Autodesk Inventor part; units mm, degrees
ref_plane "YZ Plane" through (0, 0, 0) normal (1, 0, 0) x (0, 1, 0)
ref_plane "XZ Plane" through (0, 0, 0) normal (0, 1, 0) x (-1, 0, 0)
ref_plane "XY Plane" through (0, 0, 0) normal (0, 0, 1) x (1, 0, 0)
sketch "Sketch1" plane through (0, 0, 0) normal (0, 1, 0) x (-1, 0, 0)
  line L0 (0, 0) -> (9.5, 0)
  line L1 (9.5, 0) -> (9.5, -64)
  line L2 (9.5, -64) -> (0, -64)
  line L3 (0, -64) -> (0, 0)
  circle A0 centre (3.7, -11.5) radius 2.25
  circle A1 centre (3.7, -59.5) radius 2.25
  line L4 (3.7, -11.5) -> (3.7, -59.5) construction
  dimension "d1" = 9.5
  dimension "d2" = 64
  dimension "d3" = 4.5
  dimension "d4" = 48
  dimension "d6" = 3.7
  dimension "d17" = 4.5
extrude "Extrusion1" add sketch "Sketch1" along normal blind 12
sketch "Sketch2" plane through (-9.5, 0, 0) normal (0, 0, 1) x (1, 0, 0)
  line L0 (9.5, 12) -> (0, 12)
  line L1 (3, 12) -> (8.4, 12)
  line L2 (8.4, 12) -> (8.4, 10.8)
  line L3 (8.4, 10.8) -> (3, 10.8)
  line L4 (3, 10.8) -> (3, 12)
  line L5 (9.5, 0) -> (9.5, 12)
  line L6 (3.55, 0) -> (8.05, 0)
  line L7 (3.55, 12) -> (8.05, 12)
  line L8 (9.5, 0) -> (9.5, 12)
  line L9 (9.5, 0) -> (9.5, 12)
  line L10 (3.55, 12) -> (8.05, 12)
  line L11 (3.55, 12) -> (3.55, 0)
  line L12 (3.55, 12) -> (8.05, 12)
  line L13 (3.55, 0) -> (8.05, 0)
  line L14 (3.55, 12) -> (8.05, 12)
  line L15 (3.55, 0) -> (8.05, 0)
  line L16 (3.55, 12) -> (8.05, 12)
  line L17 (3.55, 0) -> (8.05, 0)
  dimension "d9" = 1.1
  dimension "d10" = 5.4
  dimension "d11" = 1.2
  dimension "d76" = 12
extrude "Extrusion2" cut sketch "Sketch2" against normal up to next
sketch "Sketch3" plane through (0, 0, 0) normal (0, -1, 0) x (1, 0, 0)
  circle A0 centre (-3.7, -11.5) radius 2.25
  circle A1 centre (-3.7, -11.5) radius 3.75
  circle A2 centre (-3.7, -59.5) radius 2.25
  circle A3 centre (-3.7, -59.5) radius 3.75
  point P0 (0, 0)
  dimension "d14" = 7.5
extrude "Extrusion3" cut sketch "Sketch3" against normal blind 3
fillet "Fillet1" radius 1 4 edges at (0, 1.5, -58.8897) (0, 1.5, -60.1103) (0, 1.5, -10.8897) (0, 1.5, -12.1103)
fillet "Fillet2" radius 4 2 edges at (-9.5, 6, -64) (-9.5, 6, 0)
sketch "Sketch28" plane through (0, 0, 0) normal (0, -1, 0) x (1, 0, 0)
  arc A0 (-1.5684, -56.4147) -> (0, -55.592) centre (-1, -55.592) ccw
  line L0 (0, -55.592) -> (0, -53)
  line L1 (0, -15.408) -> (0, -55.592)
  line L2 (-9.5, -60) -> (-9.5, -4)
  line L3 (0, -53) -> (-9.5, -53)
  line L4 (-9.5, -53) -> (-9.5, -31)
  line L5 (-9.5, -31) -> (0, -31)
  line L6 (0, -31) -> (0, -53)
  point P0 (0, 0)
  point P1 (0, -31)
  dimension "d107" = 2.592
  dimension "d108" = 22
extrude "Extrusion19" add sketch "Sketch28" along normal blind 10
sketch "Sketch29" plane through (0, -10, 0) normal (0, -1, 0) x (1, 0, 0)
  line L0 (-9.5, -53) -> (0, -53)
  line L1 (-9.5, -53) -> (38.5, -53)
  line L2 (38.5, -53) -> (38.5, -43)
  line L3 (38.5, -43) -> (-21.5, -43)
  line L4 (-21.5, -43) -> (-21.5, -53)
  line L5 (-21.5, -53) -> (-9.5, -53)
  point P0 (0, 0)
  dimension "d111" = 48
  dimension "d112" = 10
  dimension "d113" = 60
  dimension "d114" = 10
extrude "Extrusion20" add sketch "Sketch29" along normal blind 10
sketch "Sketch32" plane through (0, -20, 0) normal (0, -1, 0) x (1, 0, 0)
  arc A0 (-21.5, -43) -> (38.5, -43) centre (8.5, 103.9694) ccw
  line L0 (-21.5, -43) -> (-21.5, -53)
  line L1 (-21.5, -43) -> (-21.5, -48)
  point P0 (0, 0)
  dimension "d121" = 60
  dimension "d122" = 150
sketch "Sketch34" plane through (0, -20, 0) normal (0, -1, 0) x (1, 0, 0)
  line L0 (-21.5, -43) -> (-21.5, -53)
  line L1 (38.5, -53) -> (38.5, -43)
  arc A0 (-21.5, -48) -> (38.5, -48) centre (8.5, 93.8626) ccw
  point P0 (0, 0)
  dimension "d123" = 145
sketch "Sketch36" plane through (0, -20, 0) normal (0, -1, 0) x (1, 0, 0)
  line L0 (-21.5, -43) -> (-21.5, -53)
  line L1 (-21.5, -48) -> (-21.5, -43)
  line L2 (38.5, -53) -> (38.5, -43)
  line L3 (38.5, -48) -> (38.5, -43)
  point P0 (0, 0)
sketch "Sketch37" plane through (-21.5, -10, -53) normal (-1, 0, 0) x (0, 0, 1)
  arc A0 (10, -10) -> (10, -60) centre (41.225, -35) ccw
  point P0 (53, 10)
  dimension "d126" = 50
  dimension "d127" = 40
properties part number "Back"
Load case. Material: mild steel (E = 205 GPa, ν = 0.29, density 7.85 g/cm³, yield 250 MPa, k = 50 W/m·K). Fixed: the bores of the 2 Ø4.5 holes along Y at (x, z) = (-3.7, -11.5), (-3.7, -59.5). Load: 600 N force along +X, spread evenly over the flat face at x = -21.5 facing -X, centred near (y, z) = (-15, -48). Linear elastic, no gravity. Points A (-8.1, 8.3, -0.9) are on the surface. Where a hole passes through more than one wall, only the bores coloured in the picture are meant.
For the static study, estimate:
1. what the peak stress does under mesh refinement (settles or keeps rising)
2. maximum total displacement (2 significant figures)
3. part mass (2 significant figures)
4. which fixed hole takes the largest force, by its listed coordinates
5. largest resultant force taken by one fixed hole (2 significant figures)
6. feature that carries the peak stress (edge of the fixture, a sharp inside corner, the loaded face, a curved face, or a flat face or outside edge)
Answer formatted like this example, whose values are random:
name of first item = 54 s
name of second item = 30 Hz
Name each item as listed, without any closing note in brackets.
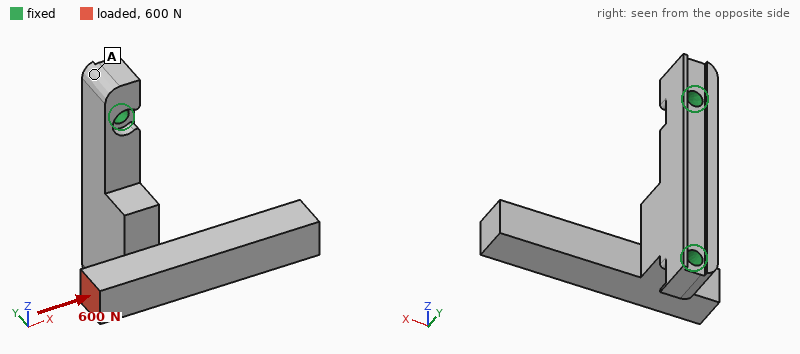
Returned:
what the peak stress does under mesh refinement = keeps rising
maximum total displacement = 63 µm
part mass = 110 g
which fixed hole takes the largest force, by its listed coordinates = (-3.7, -59.5)
largest resultant force taken by one fixed hole = 500 N
feature that carries the peak stress = edge of the fixture
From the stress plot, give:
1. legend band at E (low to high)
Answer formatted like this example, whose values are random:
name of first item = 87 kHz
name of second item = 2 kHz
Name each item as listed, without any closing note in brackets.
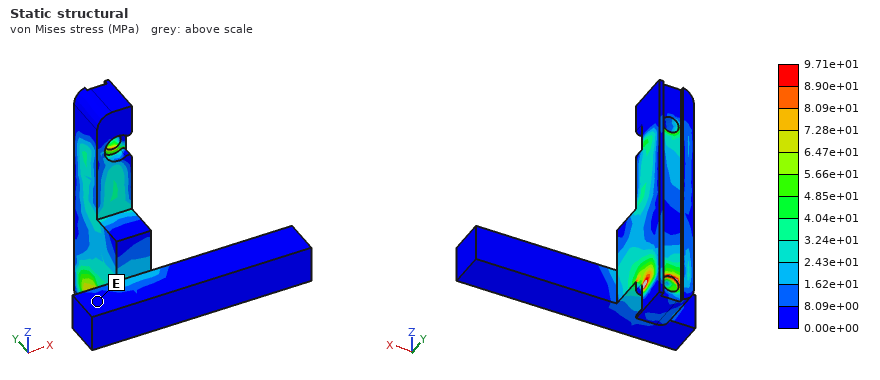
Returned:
legend band at E = 0.00e+00 to 8.09e+00 MPa
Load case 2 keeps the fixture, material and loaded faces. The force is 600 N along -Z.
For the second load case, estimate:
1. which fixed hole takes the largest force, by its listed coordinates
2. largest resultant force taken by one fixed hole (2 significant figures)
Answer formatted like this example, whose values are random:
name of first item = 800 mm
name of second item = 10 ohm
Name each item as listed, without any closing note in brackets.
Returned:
which fixed hole takes the largest force, by its listed coordinates = (-3.7, -11.5)
largest resultant force taken by one fixed hole = 540 N
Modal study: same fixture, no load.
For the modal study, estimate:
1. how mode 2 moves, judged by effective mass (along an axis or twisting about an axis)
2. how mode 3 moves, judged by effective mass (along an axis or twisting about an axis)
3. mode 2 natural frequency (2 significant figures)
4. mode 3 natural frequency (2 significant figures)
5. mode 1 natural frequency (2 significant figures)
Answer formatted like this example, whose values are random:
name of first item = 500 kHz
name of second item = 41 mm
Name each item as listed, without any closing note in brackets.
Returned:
how mode 2 moves, judged by effective mass = along Z
how mode 3 moves, judged by effective mass = along X
mode 2 natural frequency = 2900 Hz
mode 3 natural frequency = 5700 Hz
mode 1 natural frequency = 2100 Hz
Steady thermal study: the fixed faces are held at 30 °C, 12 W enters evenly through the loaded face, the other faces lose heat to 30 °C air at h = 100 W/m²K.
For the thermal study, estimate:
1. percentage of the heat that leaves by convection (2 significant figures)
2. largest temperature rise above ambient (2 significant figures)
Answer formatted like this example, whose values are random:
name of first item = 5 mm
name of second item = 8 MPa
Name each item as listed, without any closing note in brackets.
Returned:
percentage of the heat that leaves by convection = 55 %
largest temperature rise above ambient = 55 K
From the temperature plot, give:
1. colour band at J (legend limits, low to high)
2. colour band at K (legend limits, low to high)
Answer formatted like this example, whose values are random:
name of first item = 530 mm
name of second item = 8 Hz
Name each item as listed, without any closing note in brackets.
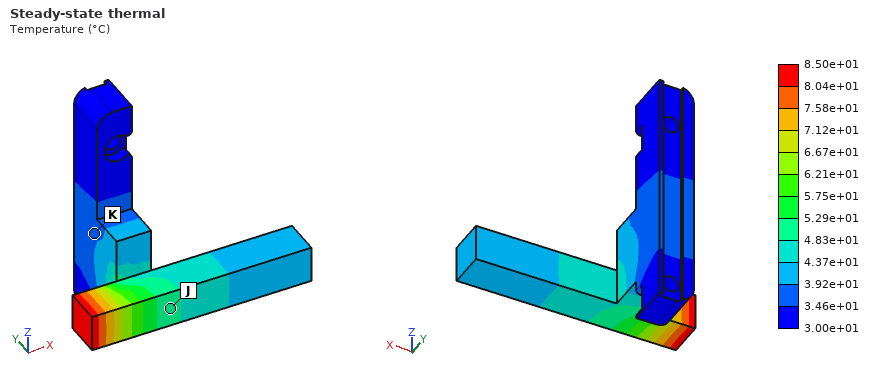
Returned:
colour band at J = 4.83e+01 to 5.29e+01 °C
colour band at K = 3.46e+01 to 3.92e+01 °C
